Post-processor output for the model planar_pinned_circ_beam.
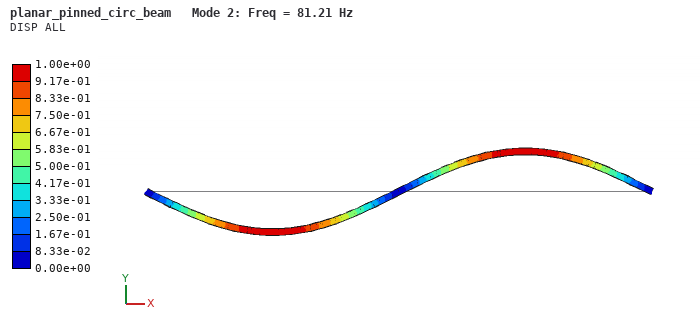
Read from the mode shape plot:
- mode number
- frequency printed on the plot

2
81.21 Hz
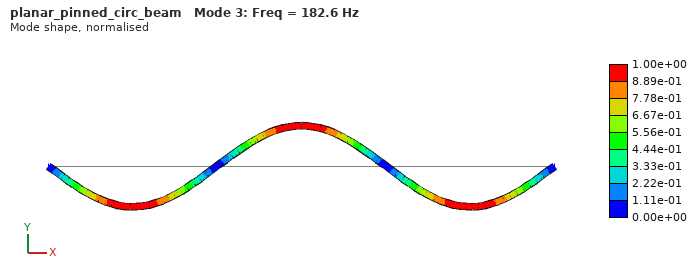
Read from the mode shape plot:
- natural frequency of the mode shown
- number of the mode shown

182.6 Hz
3
